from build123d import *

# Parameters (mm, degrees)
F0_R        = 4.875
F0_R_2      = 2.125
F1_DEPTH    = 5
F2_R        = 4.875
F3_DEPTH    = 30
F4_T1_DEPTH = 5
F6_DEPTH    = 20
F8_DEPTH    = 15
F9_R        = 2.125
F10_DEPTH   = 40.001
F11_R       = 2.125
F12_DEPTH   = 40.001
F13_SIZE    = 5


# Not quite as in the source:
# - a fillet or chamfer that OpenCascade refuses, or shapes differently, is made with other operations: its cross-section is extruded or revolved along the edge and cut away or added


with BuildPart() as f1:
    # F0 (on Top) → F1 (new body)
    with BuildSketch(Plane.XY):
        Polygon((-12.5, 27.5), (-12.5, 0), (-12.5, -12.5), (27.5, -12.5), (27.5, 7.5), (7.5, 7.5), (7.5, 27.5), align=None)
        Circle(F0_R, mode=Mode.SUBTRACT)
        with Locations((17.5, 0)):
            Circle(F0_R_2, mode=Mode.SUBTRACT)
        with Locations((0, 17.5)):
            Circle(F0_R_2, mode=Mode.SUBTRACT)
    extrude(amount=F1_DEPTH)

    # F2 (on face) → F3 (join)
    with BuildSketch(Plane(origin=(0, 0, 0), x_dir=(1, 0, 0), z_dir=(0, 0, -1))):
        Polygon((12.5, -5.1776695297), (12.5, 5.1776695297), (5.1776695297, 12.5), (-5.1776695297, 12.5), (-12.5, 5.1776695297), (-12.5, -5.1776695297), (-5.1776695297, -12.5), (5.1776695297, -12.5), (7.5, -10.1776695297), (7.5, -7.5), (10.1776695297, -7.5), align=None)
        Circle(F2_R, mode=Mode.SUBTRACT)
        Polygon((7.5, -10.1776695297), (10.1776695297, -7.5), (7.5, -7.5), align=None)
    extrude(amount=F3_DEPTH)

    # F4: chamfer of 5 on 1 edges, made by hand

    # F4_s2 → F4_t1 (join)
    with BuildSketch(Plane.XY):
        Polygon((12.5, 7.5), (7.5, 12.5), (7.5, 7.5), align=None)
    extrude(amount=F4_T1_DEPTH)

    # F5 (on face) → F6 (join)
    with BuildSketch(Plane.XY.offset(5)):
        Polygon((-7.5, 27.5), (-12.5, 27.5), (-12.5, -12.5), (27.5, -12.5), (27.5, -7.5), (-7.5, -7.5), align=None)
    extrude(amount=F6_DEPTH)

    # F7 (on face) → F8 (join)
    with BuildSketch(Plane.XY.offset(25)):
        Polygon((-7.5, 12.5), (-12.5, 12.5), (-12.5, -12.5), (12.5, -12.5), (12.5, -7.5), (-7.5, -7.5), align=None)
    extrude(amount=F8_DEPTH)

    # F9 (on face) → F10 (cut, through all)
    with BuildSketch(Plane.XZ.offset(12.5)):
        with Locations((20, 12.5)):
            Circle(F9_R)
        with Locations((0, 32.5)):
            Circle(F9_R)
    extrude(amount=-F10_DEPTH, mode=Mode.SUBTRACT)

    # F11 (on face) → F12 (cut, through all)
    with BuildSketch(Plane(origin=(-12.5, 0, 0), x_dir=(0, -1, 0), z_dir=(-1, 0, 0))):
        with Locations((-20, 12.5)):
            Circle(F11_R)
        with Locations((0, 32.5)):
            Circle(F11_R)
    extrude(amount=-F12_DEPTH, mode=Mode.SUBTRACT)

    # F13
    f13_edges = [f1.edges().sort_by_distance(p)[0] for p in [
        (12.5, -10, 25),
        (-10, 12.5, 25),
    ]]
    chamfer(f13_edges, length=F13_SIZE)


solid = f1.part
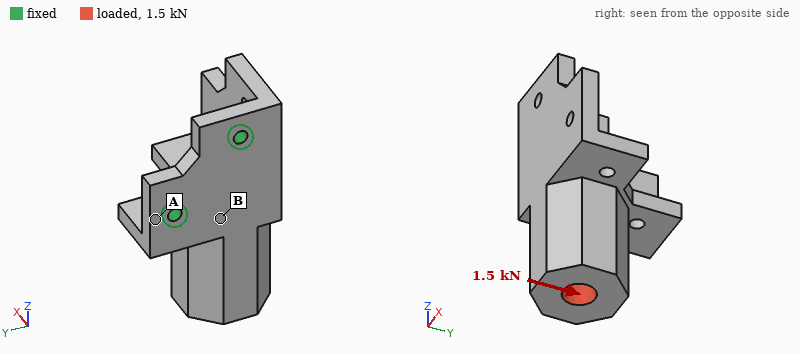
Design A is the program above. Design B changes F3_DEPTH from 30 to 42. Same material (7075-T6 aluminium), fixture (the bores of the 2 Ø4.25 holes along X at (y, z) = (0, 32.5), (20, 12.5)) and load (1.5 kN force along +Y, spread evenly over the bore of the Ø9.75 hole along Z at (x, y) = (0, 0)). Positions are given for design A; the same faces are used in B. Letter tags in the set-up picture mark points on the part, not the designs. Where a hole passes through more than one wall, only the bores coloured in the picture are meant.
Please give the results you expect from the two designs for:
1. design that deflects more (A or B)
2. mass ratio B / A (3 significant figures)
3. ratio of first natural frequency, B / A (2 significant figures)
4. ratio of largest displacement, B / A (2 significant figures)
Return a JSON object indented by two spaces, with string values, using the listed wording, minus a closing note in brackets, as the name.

{
  "design that deflects more": "B",
  "mass ratio B / A": "1.18",
  "ratio of first natural frequency, B / A": "0.79",
  "ratio of largest displacement, B / A": "1.2"
}
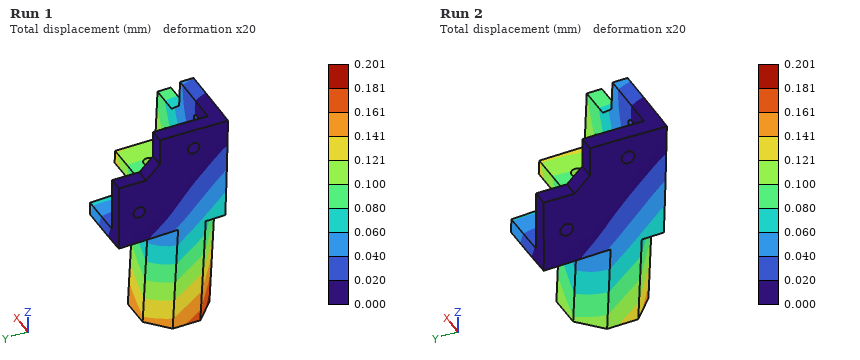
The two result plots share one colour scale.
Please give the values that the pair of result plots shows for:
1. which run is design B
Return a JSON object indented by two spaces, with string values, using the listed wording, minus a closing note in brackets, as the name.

{
  "which run is design B": "Run 1"
}
